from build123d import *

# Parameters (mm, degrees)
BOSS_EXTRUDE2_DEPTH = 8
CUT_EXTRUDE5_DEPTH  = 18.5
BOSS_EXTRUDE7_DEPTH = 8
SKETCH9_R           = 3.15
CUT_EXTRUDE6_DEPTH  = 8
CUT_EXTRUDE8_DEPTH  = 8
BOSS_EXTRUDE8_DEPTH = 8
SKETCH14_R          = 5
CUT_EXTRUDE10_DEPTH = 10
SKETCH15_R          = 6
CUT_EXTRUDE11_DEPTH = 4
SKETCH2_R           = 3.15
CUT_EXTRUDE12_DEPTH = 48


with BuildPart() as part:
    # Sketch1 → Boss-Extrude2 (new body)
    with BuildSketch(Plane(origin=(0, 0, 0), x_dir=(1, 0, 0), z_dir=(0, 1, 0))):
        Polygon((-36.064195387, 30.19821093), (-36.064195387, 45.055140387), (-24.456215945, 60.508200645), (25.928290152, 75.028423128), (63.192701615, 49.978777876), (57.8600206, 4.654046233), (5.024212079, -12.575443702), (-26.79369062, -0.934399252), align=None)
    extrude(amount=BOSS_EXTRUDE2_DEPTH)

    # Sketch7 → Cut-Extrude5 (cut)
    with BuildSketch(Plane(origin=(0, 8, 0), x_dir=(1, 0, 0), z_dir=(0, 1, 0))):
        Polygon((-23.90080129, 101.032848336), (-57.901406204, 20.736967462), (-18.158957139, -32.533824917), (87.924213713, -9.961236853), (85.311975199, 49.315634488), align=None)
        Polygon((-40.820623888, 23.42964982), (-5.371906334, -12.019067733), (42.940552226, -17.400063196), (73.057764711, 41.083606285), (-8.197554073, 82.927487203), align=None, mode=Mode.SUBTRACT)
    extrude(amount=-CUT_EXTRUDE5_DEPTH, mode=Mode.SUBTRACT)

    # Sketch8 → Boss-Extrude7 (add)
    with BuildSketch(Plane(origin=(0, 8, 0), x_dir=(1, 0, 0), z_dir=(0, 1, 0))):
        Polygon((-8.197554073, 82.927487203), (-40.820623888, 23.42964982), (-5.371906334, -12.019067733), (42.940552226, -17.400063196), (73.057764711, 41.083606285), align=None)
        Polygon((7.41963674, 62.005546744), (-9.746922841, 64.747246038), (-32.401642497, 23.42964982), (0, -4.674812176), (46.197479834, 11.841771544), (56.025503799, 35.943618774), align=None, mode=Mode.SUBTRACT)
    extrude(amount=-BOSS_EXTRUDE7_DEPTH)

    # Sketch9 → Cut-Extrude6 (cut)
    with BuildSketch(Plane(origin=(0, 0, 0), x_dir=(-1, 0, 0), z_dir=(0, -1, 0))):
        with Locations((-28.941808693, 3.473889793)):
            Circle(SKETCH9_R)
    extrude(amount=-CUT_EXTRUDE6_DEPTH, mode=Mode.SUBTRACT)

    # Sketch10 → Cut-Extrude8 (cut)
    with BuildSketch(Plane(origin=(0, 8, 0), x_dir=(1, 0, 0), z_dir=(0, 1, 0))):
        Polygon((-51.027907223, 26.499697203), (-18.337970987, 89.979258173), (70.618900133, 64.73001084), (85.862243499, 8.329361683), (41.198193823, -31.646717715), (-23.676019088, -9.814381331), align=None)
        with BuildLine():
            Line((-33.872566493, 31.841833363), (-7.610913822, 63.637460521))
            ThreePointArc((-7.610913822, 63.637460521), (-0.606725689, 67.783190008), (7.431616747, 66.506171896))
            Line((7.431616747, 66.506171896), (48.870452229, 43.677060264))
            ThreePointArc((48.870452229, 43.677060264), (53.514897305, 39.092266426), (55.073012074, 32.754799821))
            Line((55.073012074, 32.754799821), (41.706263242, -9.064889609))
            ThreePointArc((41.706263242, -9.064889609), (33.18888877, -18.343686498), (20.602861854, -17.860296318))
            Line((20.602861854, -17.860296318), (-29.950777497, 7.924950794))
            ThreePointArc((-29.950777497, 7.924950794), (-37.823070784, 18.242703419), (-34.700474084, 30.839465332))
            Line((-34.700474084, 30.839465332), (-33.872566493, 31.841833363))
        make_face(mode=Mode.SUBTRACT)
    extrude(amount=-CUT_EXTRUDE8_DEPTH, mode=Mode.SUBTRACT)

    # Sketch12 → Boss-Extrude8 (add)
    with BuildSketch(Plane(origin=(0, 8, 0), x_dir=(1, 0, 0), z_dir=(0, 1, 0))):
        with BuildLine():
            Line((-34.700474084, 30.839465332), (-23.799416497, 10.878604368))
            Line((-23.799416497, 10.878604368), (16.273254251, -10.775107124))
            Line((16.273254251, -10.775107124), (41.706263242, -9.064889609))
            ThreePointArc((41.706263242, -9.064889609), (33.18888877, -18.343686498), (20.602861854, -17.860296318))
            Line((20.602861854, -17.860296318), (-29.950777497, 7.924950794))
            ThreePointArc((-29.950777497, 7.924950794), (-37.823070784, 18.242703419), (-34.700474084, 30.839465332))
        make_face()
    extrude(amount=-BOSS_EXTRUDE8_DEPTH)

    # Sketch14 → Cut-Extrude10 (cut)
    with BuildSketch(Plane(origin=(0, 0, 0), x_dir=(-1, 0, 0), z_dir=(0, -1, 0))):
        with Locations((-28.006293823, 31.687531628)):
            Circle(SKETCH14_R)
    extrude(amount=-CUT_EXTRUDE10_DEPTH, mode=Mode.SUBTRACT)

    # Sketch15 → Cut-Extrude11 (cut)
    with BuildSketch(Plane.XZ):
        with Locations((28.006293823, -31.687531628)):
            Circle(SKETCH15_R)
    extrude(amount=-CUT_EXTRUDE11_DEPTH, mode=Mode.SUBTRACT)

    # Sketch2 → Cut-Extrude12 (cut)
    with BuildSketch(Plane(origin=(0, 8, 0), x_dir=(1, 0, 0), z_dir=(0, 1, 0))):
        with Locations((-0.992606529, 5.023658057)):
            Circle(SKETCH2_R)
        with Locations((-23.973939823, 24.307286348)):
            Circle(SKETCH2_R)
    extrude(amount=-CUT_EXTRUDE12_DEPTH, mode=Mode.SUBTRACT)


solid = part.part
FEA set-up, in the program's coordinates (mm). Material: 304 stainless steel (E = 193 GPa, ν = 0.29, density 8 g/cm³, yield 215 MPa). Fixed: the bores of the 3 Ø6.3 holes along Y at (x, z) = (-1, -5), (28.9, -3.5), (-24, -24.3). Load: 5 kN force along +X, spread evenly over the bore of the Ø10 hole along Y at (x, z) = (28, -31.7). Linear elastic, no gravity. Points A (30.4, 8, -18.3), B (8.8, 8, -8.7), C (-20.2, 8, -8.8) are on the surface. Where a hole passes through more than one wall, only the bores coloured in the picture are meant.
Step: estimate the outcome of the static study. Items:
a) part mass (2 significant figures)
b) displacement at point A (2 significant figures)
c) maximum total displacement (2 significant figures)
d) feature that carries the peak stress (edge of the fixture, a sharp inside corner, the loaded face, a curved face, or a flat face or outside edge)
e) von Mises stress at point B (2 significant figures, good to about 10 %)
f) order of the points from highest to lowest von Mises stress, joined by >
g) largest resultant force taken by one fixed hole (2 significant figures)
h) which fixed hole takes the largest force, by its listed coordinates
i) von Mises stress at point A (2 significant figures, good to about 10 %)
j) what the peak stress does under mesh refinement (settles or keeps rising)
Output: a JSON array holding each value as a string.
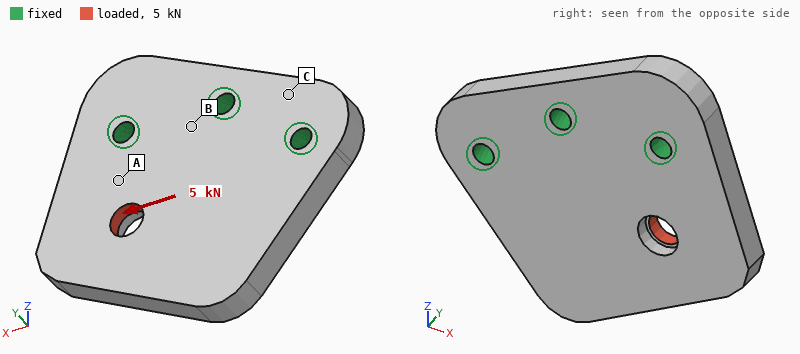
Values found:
["330 g", "3.0 µm", "12 µm", "a sharp inside corner", "13 MPa", "A > B > C", "2.7 kN", "(-24, -24.3)", "22 MPa", "keeps rising"]
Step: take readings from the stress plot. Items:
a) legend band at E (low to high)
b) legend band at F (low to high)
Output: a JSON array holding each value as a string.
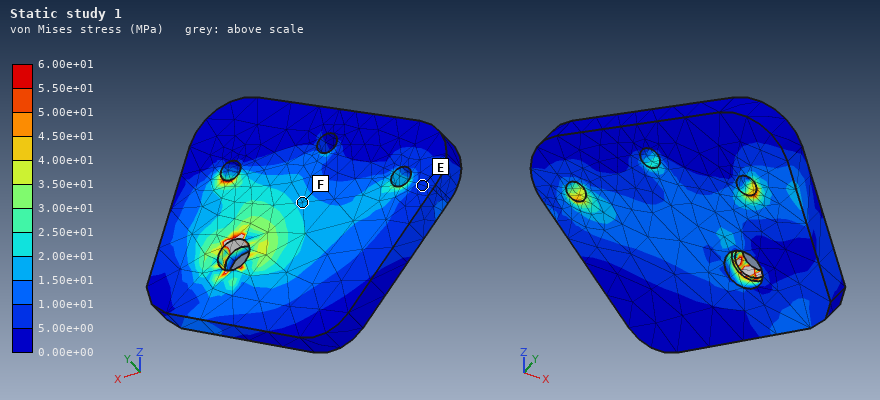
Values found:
["5.00e+00 to 1.00e+01 MPa", "1.50e+01 to 2.00e+01 MPa"]
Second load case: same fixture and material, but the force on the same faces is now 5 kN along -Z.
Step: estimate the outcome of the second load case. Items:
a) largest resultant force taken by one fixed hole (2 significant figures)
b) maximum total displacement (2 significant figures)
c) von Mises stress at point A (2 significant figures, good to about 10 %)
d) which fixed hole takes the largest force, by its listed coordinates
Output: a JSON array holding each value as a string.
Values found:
["4.1 kN", "17 µm", "39 MPa", "(28.9, -3.5)"]
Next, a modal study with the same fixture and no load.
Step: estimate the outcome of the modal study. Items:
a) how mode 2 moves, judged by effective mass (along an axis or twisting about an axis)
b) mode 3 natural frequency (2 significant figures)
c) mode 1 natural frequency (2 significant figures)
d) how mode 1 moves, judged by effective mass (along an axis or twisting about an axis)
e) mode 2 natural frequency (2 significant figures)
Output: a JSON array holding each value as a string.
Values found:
["twisting about Z", "11 kHz", "2700 Hz", "along Y", "5400 Hz"]
